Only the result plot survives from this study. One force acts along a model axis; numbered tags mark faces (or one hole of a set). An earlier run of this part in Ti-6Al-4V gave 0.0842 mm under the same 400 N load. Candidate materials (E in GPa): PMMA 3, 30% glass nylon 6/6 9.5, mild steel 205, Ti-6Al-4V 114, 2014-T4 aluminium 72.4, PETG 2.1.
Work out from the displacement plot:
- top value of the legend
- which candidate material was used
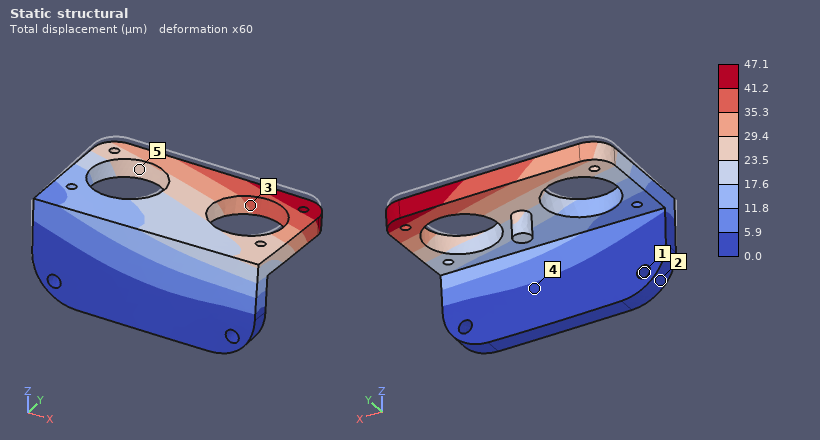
47.1 µm
mild steel
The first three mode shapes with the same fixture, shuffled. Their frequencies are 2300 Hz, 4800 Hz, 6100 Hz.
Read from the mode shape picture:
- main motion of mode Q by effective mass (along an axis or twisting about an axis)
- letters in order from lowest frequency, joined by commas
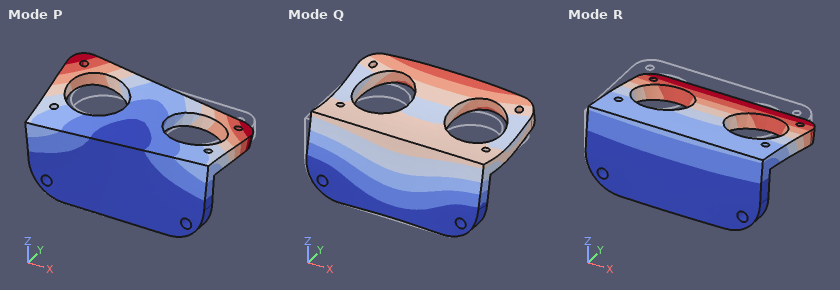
along Y
R, P, Q
